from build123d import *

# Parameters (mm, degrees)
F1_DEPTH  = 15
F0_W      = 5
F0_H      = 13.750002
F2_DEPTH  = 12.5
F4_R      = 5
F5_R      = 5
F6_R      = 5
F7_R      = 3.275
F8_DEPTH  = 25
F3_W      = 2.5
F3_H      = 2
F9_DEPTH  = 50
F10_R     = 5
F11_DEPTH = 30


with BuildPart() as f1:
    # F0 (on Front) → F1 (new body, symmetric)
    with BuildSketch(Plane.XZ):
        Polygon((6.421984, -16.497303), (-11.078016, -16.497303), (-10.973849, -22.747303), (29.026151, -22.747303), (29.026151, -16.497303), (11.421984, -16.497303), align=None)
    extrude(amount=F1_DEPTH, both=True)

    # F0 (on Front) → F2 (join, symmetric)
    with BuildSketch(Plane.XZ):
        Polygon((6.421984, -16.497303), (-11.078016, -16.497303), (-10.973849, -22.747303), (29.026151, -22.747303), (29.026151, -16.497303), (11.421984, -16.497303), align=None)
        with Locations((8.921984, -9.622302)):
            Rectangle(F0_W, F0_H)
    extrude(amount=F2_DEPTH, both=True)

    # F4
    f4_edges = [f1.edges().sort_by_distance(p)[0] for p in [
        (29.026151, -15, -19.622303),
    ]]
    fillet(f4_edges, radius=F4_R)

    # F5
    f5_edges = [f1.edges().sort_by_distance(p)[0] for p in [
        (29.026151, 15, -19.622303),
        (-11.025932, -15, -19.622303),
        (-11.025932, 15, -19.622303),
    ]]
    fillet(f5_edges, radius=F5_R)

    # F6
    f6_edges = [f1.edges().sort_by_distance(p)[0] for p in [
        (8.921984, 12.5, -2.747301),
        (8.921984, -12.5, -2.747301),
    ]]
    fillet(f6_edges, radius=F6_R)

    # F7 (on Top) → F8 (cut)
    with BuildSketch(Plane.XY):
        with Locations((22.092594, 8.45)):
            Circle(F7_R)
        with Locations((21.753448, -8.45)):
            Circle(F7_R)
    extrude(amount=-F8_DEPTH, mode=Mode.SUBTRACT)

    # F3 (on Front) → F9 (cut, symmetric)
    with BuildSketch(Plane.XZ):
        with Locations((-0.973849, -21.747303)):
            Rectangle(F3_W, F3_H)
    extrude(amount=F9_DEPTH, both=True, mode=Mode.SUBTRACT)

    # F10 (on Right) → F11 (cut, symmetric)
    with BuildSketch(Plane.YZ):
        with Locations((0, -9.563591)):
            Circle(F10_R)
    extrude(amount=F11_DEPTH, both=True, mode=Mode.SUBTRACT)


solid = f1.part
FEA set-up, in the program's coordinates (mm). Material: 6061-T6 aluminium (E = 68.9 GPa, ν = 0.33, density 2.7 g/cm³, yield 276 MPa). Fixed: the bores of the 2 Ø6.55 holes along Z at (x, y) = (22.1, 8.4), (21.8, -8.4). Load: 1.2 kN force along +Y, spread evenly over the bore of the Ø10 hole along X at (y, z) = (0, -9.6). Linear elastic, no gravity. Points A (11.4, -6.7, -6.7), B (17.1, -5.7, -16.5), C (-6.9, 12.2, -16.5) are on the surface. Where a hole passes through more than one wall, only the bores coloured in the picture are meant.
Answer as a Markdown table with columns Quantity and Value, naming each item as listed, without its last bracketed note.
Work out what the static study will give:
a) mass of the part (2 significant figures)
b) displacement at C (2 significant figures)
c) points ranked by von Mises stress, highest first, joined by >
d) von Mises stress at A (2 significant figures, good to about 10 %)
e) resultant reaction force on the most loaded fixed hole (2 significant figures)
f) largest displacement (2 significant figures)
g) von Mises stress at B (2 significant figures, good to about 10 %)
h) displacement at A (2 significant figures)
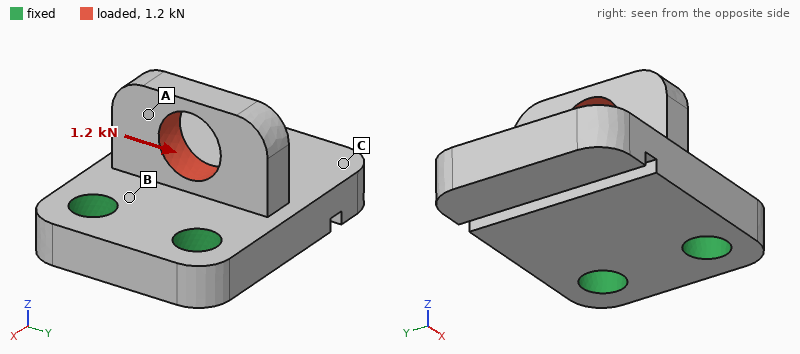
| Quantity | Value |
|---|---|
| mass of the part | 22 g |
| displacement at C | 17 µm |
| points ranked by von Mises stress, highest first, joined by > | B > A > C |
| von Mises stress at A | 23 MPa |
| resultant reaction force on the most loaded fixed hole | 1.0 kN |
| largest displacement | 31 µm |
| von Mises stress at B | 32 MPa |
| displacement at A | 24 µm |
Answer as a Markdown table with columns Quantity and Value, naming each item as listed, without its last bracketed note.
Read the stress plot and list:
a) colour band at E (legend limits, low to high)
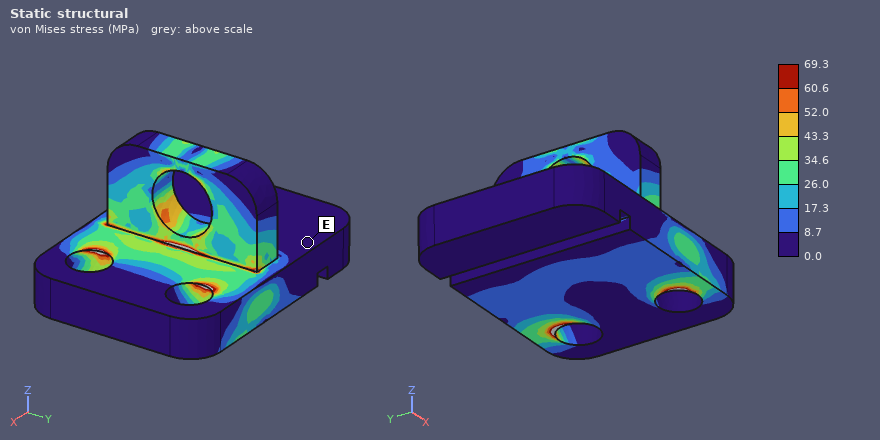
| Quantity | Value |
|---|---|
| colour band at E | 0.0 to 8.7 MPa |
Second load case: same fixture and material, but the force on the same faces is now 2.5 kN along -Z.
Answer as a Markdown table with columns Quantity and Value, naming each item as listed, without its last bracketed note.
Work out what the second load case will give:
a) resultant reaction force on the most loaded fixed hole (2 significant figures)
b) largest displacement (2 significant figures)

| Quantity | Value |
|---|---|
| resultant reaction force on the most loaded fixed hole | 1.3 kN |
| largest displacement | 0.11 mm |
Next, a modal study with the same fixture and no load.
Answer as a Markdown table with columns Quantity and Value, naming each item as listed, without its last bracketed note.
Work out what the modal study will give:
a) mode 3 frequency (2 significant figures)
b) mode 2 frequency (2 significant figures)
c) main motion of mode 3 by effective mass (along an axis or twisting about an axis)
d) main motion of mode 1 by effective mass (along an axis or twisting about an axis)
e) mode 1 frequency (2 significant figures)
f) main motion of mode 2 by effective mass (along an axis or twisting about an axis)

| Quantity | Value |
|---|---|
| mode 3 frequency | 16 kHz |
| mode 2 frequency | 11 kHz |
| main motion of mode 3 by effective mass | along Y |
| main motion of mode 1 by effective mass | along Z |
| mode 1 frequency | 5100 Hz |
| main motion of mode 2 by effective mass | twisting about X |
